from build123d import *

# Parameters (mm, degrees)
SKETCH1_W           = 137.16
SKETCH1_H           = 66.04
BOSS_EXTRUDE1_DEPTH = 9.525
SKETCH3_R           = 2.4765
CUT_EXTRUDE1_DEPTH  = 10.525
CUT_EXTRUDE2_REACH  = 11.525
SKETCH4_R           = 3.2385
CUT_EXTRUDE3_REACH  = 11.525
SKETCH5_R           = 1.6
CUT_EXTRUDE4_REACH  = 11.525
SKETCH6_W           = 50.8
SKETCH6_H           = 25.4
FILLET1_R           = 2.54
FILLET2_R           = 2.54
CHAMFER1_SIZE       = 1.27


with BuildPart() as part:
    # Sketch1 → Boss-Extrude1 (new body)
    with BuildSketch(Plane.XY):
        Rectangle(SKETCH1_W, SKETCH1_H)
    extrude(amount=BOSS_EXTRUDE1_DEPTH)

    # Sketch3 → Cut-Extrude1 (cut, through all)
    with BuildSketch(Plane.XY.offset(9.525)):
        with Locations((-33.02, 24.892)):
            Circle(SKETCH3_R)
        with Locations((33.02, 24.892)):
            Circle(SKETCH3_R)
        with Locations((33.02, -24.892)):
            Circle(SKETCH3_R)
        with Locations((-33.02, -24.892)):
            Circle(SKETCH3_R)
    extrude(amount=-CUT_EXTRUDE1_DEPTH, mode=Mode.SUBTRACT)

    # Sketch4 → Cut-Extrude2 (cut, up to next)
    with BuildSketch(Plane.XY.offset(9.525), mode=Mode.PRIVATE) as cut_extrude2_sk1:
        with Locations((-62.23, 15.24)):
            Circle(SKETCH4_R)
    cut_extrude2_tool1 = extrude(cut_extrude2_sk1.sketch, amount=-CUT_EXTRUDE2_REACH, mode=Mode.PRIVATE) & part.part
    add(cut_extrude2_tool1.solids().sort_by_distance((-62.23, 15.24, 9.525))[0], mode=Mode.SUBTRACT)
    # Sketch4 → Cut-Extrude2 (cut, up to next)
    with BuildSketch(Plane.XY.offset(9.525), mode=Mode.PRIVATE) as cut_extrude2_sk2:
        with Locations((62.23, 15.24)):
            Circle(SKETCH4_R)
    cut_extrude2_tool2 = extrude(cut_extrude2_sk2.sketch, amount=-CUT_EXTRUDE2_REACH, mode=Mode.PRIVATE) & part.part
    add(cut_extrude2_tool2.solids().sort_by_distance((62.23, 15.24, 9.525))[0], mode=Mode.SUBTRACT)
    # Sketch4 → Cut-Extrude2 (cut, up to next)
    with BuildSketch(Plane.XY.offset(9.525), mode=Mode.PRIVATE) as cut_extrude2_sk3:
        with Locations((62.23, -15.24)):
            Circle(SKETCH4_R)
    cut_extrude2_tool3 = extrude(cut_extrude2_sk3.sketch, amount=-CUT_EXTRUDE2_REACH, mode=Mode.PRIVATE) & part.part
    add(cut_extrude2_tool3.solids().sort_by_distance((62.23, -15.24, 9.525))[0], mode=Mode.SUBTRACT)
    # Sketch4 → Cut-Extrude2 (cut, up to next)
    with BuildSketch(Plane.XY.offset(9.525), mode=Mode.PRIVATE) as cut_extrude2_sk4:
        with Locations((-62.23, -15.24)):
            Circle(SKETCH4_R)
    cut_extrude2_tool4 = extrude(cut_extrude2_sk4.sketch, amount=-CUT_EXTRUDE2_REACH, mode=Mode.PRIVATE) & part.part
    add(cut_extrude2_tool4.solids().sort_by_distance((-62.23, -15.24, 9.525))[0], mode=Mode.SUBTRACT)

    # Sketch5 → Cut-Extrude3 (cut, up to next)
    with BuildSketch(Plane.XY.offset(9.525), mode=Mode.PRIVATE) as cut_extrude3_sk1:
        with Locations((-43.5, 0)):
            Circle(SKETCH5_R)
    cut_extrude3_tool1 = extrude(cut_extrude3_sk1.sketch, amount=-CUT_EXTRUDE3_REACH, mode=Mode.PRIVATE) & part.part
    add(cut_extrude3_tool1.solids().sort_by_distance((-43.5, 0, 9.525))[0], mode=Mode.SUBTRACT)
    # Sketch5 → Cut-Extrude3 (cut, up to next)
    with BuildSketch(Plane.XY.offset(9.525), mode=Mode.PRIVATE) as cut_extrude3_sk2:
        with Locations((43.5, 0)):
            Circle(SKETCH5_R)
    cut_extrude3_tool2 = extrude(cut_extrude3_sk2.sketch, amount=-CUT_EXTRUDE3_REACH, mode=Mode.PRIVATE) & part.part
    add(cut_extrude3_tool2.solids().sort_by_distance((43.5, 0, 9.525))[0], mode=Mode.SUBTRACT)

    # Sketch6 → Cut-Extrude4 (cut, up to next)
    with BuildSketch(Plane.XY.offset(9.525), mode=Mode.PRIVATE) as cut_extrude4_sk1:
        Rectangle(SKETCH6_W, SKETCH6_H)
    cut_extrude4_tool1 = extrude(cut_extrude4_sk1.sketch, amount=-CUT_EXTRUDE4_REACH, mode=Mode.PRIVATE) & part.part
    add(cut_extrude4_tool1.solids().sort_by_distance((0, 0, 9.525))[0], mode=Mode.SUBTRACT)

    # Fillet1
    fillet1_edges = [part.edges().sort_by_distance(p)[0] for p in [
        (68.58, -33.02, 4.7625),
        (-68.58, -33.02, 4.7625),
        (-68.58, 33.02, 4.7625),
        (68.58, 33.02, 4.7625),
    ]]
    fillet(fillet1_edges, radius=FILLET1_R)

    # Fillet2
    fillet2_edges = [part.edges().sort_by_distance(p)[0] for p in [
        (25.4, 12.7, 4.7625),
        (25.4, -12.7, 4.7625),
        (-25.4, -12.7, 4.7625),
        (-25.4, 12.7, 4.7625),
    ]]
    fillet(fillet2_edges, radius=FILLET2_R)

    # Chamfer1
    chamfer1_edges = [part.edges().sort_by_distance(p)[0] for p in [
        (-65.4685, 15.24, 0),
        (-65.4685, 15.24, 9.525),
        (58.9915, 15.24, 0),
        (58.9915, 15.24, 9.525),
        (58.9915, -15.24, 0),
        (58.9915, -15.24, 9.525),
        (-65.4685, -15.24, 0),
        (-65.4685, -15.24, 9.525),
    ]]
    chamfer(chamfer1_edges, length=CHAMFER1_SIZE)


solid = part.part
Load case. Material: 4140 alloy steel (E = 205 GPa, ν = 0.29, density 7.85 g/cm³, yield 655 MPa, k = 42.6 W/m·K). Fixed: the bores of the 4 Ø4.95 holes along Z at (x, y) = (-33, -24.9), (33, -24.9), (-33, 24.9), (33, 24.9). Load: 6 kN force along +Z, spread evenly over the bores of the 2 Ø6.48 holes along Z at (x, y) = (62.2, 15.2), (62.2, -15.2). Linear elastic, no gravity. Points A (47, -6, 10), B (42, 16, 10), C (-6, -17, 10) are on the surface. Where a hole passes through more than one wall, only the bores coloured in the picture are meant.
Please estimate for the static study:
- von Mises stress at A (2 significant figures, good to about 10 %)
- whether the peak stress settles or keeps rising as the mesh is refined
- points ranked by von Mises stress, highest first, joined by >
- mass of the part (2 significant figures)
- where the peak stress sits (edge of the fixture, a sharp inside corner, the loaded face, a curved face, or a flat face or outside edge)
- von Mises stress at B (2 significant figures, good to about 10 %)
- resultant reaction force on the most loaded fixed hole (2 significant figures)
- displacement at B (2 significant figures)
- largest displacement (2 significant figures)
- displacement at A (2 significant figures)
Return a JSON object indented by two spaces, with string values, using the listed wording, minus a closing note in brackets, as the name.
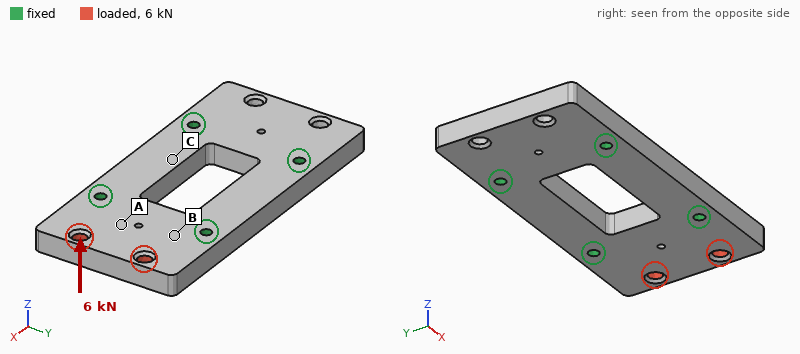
{
  "von Mises stress at A": "84 MPa",
  "whether the peak stress settles or keeps rising as the mesh is refined": "keeps rising",
  "points ranked by von Mises stress, highest first, joined by >": "B > A > C",
  "mass of the part": "560 g",
  "where the peak stress sits": "edge of the fixture",
  "von Mises stress at B": "120 MPa",
  "resultant reaction force on the most loaded fixed hole": "3.3 kN",
  "displacement at B": "0.021 mm",
  "largest displacement": "0.11 mm",
  "displacement at A": "0.038 mm"
}
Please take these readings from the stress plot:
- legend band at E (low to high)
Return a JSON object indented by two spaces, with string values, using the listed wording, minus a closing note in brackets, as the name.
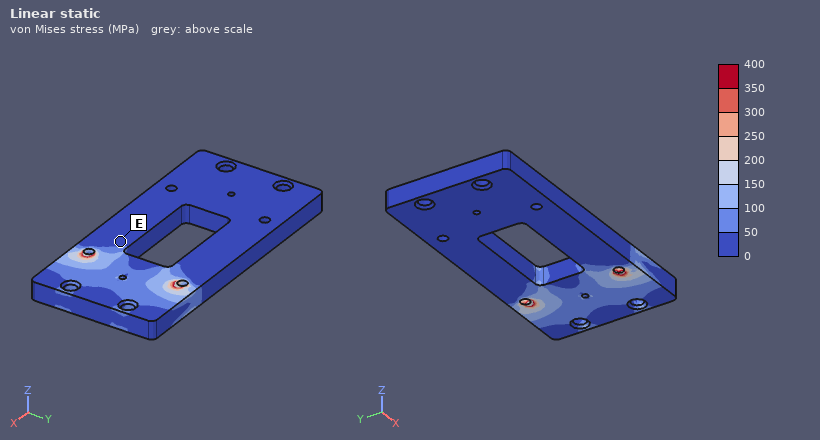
{
  "legend band at E": "0 to 50 MPa"
}
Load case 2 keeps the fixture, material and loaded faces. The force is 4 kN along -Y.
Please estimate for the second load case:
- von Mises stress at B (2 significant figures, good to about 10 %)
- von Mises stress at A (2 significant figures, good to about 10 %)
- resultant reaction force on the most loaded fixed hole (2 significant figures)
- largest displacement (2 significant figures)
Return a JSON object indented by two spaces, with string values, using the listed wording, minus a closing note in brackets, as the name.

{
  "von Mises stress at B": "16 MPa",
  "von Mises stress at A": "14 MPa",
  "resultant reaction force on the most loaded fixed hole": "2.9 kN",
  "largest displacement": "5.0 µm"
}
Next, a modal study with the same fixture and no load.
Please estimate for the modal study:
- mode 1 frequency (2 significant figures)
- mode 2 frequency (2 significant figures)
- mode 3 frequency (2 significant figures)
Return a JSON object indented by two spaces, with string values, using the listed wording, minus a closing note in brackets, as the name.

{
  "mode 1 frequency": "4900 Hz",
  "mode 2 frequency": "5000 Hz",
  "mode 3 frequency": "8900 Hz"
}
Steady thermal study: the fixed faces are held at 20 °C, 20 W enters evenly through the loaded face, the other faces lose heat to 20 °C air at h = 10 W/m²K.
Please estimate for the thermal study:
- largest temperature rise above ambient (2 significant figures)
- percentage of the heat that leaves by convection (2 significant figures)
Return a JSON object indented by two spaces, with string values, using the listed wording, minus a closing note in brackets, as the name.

{
  "largest temperature rise above ambient": "32 K",
  "percentage of the heat that leaves by convection": "5.9 %"
}
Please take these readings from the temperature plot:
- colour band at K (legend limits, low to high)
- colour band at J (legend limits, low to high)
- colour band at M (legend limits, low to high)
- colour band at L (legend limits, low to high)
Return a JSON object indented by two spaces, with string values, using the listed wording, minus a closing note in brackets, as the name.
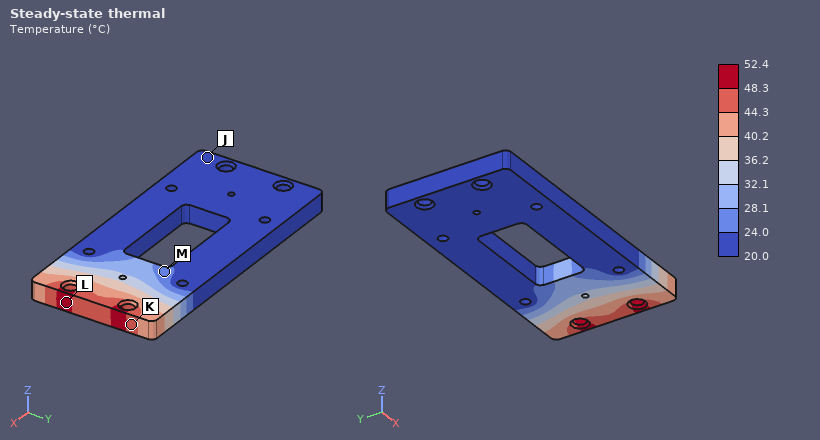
{
  "colour band at K": "44.3 to 48.3 °C",
  "colour band at J": "20.0 to 24.0 °C",
  "colour band at M": "24.0 to 28.1 °C",
  "colour band at L": "48.3 to 52.4 °C"
}
